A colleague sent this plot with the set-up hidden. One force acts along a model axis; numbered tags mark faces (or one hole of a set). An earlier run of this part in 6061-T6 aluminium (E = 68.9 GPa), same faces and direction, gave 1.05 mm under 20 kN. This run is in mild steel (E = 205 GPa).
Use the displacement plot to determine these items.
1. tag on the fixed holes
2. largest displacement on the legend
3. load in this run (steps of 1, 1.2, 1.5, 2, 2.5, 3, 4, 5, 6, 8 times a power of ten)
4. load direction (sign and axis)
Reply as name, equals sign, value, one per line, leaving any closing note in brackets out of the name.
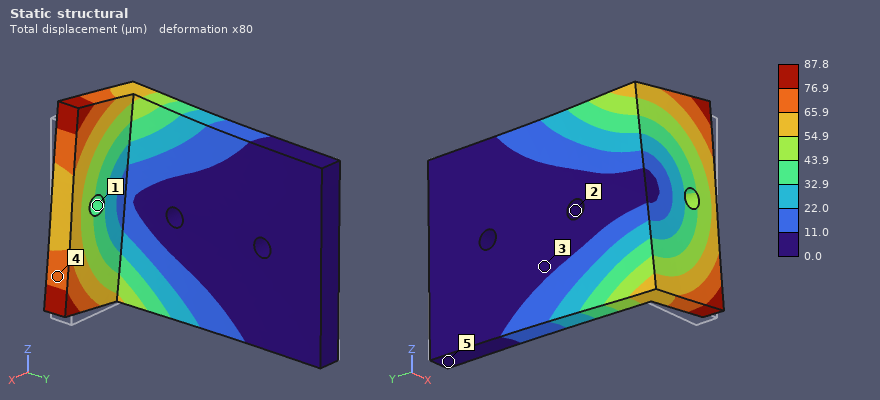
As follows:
tag on the fixed holes = 2
largest displacement on the legend = 87.8 µm
load in this run = 5 kN
load direction = +Z
